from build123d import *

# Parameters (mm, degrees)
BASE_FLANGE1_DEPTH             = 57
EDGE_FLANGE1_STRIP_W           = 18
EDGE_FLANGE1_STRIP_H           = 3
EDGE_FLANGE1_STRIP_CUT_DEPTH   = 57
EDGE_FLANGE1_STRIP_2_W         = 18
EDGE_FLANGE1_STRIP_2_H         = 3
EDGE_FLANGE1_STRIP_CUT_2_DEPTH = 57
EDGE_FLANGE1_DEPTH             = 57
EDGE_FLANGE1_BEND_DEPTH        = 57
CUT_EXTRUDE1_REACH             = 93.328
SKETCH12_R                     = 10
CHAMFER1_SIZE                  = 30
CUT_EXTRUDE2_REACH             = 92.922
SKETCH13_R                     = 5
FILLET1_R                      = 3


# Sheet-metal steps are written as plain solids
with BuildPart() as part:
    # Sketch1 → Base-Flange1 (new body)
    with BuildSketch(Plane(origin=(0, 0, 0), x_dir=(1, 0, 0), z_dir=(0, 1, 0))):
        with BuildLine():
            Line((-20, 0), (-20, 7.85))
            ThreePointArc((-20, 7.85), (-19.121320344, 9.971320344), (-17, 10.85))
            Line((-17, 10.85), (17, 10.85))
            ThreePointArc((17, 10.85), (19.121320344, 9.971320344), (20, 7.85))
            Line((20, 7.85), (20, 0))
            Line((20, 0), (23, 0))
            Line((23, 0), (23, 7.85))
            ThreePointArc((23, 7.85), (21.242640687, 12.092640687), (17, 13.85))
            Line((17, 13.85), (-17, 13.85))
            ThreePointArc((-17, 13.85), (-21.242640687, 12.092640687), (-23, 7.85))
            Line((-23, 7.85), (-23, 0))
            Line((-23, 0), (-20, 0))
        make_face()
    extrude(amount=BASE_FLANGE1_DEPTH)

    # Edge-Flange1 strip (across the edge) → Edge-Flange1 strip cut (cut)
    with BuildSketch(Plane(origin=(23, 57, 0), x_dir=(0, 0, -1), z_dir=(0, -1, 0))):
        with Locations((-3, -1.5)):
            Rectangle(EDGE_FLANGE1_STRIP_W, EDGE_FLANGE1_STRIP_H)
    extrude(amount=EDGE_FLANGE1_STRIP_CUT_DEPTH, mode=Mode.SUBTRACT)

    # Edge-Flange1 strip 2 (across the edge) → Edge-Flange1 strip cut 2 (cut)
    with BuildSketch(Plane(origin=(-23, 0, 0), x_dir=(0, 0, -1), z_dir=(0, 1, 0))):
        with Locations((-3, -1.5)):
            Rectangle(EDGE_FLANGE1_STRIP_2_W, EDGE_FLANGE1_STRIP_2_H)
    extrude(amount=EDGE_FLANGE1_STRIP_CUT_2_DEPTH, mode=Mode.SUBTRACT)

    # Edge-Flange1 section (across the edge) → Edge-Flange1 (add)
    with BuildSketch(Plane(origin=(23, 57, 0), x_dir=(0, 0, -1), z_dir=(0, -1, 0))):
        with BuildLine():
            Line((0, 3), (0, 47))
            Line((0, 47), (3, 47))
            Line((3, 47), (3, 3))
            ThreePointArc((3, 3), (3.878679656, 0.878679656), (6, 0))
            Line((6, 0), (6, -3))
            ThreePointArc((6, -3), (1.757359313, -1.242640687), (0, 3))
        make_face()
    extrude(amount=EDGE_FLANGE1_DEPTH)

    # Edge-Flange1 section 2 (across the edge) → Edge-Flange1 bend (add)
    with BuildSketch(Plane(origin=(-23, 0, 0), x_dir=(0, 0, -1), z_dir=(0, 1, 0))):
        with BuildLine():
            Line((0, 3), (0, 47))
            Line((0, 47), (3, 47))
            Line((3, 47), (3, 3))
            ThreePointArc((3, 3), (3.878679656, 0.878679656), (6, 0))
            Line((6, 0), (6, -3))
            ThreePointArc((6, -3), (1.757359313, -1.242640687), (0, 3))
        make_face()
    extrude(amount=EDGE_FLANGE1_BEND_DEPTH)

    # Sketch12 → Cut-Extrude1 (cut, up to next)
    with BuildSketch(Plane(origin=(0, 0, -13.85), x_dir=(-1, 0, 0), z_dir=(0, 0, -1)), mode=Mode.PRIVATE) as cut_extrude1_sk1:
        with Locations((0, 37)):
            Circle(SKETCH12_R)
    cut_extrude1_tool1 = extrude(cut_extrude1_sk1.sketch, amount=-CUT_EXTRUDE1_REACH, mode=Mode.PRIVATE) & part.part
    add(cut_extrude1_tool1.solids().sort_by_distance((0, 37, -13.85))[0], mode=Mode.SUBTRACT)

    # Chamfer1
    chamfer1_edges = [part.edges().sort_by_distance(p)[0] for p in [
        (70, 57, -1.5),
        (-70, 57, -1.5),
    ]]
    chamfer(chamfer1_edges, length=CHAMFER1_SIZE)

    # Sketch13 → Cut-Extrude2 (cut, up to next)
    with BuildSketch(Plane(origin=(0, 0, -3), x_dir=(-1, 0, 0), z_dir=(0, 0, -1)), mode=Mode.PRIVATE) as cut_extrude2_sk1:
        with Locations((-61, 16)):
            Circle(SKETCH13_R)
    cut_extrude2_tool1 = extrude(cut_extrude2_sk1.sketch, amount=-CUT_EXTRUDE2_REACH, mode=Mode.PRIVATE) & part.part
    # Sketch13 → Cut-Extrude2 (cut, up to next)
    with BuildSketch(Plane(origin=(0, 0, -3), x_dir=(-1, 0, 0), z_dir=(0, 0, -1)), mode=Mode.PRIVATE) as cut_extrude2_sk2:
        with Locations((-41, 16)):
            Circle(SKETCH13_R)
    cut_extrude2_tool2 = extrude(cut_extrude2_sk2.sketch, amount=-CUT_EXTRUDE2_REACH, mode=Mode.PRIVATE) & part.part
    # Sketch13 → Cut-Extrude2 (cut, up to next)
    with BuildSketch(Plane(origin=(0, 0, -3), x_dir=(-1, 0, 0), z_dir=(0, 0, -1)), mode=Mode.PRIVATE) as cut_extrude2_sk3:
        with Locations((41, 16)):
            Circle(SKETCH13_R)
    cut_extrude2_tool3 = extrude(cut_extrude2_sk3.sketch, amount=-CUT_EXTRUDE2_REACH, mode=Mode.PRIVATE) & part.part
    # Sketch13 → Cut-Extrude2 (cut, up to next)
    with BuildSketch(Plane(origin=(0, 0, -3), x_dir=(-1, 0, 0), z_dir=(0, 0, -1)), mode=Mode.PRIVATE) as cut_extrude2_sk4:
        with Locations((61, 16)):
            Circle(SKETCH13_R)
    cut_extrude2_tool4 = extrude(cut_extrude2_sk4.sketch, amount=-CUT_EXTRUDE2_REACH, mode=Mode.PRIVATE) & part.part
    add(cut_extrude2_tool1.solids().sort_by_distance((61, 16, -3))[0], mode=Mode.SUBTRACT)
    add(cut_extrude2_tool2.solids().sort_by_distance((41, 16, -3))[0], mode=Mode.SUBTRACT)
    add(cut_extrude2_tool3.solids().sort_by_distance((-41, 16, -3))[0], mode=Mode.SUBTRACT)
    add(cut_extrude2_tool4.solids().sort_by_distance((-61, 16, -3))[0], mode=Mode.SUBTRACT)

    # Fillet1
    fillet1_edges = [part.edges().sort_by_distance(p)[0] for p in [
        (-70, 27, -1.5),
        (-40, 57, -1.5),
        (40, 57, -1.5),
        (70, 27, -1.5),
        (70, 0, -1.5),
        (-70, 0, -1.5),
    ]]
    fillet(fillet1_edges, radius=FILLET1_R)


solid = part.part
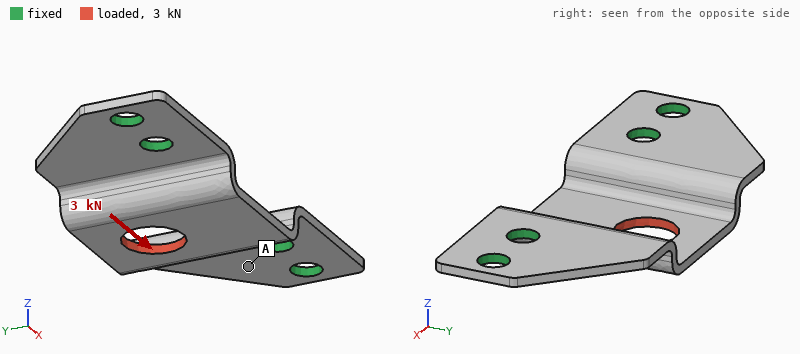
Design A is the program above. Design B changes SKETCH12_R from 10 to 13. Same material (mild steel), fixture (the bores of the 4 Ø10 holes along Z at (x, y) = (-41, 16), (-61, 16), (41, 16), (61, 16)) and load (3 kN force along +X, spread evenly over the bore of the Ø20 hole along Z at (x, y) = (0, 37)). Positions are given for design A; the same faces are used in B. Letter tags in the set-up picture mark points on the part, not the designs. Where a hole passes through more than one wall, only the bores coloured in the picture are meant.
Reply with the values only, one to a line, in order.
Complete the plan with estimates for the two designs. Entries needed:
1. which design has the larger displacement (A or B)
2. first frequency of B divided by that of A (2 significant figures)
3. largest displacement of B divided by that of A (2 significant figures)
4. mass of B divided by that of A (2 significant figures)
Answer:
B
1.0
1.2
0.97
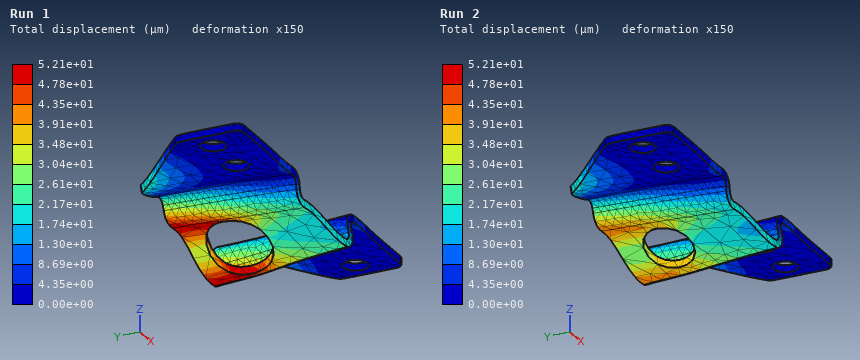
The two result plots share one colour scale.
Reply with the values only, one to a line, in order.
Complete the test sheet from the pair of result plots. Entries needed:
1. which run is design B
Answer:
Run 1
